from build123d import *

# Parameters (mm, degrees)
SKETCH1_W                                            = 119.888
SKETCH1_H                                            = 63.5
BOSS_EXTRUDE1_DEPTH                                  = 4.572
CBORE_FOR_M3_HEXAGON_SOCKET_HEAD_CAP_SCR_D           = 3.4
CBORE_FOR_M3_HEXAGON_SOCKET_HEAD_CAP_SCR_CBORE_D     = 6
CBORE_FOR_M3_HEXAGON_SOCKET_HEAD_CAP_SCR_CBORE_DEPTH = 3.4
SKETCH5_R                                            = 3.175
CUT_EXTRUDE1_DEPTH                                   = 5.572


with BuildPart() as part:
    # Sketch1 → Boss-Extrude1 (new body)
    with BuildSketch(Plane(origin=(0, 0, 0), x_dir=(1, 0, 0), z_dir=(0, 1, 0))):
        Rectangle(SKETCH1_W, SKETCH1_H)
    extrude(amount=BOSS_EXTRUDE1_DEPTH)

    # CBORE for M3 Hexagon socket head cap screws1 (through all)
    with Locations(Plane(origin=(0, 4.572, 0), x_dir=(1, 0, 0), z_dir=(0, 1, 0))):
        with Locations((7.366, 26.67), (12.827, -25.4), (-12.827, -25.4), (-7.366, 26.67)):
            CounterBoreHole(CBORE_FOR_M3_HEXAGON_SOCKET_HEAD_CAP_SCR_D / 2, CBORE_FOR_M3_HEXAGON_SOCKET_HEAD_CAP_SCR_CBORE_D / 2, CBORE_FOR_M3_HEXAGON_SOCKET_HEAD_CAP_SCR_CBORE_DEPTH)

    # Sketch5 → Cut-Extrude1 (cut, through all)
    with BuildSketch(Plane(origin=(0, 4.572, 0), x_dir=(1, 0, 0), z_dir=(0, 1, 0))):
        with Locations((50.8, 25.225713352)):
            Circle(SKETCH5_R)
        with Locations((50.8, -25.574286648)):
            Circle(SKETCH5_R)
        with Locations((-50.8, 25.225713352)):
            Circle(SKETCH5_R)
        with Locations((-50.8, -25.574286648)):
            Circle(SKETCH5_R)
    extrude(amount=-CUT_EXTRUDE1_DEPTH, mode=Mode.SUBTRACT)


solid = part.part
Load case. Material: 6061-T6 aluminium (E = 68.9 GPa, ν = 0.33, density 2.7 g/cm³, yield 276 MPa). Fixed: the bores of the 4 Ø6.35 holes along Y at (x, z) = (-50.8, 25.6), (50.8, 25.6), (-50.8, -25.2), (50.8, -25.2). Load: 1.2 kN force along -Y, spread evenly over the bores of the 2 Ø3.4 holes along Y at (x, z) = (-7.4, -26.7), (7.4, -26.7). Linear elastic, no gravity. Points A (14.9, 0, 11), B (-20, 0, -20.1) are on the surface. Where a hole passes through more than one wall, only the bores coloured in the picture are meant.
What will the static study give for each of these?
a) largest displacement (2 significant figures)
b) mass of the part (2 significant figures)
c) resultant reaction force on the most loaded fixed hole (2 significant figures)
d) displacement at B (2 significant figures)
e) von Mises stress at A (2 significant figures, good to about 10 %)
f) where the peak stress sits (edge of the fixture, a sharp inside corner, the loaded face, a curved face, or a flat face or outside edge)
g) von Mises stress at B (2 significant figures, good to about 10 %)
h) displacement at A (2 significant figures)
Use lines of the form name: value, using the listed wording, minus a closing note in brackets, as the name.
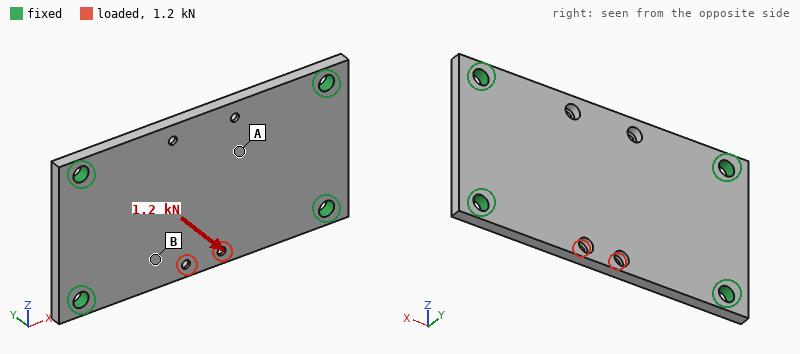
largest displacement: 0.47 mm
mass of the part: 91 g
resultant reaction force on the most loaded fixed hole: 630 N
displacement at B: 0.23 mm
von Mises stress at A: 28 MPa
where the peak stress sits: the loaded face
von Mises stress at B: 70 MPa
displacement at A: 0.099 mm
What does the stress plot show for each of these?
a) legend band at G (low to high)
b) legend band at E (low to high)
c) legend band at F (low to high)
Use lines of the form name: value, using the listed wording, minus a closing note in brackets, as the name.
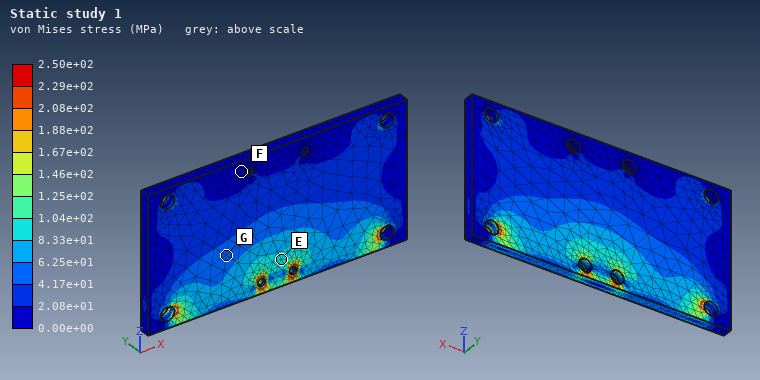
legend band at G: 4.17e+01 to 6.25e+01 MPa
legend band at E: 8.33e+01 to 1.04e+02 MPa
legend band at F: 0.00e+00 to 2.08e+01 MPa
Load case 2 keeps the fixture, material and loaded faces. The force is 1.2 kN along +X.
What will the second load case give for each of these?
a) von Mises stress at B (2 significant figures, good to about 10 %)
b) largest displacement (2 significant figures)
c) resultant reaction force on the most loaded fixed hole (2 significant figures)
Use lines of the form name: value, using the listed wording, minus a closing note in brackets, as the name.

von Mises stress at B: 8.4 MPa
largest displacement: 8.9 µm
resultant reaction force on the most loaded fixed hole: 420 N
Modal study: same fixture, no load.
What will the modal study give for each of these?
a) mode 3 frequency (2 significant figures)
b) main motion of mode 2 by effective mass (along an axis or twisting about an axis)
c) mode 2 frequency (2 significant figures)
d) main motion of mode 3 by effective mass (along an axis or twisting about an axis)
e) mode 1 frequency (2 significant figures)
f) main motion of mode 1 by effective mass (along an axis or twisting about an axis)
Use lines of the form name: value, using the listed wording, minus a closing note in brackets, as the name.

mode 3 frequency: 5800 Hz
main motion of mode 2 by effective mass: twisting about X
mode 2 frequency: 3500 Hz
main motion of mode 3 by effective mass: twisting about Z
mode 1 frequency: 2200 Hz
main motion of mode 1 by effective mass: along Y
